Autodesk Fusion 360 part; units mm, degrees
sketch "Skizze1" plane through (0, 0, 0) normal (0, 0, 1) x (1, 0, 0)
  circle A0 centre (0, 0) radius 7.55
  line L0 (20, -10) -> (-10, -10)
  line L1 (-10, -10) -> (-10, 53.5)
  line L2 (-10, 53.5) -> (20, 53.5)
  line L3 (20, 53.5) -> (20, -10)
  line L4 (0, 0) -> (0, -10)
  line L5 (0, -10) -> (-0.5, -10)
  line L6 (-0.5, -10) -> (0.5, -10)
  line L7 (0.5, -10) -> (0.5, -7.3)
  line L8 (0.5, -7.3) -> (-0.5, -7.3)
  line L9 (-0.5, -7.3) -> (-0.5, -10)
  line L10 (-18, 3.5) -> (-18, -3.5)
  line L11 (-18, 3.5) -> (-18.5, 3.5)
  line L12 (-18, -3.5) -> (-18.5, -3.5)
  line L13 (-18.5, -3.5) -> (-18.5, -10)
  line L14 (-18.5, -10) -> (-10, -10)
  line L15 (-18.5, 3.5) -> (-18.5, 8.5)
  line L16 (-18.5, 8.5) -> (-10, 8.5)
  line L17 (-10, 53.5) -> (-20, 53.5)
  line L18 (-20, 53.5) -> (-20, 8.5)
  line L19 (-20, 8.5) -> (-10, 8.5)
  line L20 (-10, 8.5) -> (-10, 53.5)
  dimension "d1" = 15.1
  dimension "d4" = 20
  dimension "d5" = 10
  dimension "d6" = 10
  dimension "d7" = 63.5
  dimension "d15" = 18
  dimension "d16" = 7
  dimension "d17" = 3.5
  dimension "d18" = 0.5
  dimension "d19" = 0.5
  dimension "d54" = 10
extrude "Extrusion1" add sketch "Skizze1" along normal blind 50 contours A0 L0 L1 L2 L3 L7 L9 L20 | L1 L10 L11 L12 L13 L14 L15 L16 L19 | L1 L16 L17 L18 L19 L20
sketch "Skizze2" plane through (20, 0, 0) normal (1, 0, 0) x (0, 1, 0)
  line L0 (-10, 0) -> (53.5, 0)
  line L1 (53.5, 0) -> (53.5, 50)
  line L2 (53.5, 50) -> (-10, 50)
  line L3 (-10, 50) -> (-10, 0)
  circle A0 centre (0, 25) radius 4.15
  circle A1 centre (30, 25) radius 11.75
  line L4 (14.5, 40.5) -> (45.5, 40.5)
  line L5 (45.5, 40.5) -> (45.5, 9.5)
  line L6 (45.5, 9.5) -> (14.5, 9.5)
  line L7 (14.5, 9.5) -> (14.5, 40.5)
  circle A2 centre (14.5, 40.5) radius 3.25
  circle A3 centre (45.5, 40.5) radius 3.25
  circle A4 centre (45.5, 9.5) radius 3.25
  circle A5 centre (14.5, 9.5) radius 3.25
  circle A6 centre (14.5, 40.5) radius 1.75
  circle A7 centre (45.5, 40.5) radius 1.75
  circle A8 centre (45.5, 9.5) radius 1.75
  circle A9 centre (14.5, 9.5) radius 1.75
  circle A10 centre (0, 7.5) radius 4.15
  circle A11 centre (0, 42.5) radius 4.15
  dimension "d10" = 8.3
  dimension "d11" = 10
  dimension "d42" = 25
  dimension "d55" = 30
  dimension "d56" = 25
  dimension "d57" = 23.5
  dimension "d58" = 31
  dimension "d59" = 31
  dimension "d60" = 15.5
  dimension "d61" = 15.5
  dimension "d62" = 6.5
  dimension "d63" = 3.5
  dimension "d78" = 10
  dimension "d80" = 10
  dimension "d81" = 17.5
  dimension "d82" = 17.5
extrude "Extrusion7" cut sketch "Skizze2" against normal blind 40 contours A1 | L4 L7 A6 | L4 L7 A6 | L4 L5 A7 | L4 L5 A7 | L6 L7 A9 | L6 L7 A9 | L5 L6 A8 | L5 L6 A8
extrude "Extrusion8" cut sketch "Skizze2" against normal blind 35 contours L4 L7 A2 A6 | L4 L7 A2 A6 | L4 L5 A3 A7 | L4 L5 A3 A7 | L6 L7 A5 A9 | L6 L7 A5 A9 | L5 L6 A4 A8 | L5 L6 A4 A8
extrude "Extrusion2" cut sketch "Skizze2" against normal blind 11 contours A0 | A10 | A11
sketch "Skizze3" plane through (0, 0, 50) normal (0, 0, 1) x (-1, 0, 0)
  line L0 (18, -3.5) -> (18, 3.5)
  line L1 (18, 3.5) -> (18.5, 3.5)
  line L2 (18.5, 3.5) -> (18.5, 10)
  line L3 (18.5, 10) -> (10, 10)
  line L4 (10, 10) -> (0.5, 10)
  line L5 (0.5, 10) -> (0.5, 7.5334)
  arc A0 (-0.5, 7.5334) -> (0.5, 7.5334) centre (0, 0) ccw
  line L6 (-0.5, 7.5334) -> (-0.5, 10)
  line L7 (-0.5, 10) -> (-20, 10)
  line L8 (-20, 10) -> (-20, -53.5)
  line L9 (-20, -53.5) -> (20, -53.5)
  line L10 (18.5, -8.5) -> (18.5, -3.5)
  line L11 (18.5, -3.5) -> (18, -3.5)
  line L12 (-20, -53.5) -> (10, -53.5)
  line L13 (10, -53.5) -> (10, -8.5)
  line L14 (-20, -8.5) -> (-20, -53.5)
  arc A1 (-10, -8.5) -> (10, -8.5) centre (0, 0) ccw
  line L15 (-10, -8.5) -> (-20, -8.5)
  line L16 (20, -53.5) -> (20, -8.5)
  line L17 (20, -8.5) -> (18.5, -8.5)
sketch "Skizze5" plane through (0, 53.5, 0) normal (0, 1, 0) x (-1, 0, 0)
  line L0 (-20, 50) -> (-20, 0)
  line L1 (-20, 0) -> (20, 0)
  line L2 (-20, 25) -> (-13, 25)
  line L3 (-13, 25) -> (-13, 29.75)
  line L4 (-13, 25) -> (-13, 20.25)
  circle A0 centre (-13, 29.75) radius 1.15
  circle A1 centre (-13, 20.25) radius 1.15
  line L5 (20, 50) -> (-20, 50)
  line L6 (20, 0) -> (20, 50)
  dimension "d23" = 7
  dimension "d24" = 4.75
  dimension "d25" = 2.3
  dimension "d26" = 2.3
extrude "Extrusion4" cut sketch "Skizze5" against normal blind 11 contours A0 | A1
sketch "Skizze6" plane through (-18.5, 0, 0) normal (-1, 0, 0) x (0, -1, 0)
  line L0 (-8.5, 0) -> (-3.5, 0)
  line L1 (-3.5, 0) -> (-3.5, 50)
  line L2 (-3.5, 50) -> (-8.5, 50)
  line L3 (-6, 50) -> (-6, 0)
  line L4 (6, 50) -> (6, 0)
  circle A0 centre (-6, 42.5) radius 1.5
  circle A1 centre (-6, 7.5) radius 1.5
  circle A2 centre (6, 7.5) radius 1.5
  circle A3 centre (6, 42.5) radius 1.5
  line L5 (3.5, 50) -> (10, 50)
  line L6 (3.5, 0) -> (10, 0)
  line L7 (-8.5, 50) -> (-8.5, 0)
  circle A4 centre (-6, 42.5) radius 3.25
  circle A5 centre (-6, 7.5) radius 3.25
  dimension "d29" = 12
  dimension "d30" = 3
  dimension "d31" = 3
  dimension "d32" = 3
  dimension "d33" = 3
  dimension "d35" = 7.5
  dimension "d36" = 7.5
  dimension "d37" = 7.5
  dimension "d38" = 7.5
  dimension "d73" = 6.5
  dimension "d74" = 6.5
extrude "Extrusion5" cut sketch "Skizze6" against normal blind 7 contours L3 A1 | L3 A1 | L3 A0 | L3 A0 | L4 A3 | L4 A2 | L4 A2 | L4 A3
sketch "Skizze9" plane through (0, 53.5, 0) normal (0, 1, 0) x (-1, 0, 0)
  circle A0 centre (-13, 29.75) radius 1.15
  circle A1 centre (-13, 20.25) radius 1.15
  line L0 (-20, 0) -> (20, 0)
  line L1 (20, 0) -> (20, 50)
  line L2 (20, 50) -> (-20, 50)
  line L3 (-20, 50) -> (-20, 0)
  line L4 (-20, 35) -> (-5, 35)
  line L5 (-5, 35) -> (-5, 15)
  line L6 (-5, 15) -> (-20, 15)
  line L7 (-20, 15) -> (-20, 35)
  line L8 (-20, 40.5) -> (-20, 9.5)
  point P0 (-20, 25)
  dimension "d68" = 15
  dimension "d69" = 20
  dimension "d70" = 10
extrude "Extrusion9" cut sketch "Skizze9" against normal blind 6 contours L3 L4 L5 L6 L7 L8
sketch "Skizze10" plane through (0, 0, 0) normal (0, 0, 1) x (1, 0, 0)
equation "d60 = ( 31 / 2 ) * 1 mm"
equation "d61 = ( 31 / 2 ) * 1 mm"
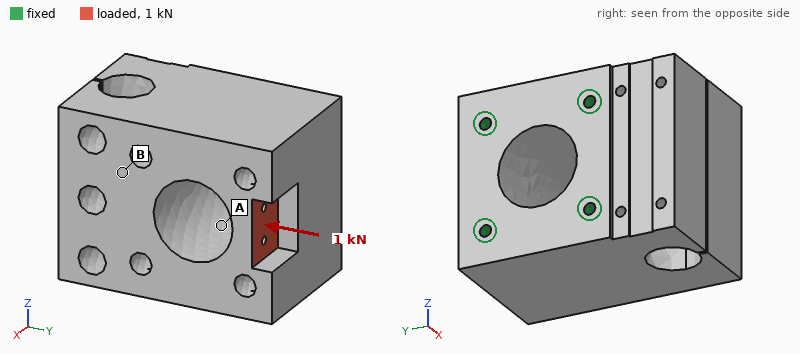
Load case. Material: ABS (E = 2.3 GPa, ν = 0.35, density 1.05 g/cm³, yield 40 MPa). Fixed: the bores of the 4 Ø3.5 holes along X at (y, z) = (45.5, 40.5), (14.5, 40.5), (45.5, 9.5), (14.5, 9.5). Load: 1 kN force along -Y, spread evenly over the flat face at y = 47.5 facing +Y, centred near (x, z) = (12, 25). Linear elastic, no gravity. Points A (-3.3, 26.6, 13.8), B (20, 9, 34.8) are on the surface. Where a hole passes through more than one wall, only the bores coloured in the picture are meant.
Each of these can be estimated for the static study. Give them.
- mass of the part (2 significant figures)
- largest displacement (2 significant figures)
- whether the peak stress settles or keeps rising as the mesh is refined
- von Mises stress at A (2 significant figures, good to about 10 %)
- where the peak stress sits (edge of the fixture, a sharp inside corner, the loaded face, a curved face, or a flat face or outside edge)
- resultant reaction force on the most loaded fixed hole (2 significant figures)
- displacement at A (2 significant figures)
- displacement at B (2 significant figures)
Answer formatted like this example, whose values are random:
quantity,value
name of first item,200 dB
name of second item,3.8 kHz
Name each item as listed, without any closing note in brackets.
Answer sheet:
quantity,value
mass of the part,95 g
largest displacement,0.23 mm
whether the peak stress settles or keeps rising as the mesh is refined,keeps rising
von Mises stress at A,2.8 MPa
where the peak stress sits,edge of the fixture
resultant reaction force on the most loaded fixed hole,520 N
displacement at A,0.048 mm
displacement at B,0.11 mm
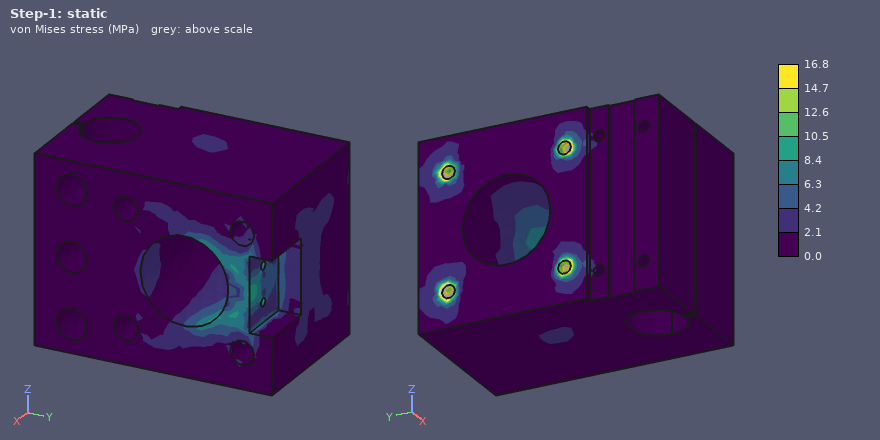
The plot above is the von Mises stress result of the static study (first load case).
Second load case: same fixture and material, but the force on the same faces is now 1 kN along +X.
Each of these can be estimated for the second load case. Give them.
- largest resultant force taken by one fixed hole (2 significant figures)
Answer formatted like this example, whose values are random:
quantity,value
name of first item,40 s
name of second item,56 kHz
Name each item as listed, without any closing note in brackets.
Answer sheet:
quantity,value
largest resultant force taken by one fixed hole,530 N
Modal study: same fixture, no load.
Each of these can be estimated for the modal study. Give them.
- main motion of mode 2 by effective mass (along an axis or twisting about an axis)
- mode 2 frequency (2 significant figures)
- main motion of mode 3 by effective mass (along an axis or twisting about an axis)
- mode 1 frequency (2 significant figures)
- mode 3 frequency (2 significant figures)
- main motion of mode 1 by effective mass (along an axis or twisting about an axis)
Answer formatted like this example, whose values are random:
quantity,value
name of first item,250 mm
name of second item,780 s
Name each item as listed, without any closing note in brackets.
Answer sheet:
quantity,value
main motion of mode 2 by effective mass,along Z
mode 2 frequency,2000 Hz
main motion of mode 3 by effective mass,twisting about X
mode 1 frequency,1800 Hz
mode 3 frequency,3300 Hz
main motion of mode 1 by effective mass,along Y
